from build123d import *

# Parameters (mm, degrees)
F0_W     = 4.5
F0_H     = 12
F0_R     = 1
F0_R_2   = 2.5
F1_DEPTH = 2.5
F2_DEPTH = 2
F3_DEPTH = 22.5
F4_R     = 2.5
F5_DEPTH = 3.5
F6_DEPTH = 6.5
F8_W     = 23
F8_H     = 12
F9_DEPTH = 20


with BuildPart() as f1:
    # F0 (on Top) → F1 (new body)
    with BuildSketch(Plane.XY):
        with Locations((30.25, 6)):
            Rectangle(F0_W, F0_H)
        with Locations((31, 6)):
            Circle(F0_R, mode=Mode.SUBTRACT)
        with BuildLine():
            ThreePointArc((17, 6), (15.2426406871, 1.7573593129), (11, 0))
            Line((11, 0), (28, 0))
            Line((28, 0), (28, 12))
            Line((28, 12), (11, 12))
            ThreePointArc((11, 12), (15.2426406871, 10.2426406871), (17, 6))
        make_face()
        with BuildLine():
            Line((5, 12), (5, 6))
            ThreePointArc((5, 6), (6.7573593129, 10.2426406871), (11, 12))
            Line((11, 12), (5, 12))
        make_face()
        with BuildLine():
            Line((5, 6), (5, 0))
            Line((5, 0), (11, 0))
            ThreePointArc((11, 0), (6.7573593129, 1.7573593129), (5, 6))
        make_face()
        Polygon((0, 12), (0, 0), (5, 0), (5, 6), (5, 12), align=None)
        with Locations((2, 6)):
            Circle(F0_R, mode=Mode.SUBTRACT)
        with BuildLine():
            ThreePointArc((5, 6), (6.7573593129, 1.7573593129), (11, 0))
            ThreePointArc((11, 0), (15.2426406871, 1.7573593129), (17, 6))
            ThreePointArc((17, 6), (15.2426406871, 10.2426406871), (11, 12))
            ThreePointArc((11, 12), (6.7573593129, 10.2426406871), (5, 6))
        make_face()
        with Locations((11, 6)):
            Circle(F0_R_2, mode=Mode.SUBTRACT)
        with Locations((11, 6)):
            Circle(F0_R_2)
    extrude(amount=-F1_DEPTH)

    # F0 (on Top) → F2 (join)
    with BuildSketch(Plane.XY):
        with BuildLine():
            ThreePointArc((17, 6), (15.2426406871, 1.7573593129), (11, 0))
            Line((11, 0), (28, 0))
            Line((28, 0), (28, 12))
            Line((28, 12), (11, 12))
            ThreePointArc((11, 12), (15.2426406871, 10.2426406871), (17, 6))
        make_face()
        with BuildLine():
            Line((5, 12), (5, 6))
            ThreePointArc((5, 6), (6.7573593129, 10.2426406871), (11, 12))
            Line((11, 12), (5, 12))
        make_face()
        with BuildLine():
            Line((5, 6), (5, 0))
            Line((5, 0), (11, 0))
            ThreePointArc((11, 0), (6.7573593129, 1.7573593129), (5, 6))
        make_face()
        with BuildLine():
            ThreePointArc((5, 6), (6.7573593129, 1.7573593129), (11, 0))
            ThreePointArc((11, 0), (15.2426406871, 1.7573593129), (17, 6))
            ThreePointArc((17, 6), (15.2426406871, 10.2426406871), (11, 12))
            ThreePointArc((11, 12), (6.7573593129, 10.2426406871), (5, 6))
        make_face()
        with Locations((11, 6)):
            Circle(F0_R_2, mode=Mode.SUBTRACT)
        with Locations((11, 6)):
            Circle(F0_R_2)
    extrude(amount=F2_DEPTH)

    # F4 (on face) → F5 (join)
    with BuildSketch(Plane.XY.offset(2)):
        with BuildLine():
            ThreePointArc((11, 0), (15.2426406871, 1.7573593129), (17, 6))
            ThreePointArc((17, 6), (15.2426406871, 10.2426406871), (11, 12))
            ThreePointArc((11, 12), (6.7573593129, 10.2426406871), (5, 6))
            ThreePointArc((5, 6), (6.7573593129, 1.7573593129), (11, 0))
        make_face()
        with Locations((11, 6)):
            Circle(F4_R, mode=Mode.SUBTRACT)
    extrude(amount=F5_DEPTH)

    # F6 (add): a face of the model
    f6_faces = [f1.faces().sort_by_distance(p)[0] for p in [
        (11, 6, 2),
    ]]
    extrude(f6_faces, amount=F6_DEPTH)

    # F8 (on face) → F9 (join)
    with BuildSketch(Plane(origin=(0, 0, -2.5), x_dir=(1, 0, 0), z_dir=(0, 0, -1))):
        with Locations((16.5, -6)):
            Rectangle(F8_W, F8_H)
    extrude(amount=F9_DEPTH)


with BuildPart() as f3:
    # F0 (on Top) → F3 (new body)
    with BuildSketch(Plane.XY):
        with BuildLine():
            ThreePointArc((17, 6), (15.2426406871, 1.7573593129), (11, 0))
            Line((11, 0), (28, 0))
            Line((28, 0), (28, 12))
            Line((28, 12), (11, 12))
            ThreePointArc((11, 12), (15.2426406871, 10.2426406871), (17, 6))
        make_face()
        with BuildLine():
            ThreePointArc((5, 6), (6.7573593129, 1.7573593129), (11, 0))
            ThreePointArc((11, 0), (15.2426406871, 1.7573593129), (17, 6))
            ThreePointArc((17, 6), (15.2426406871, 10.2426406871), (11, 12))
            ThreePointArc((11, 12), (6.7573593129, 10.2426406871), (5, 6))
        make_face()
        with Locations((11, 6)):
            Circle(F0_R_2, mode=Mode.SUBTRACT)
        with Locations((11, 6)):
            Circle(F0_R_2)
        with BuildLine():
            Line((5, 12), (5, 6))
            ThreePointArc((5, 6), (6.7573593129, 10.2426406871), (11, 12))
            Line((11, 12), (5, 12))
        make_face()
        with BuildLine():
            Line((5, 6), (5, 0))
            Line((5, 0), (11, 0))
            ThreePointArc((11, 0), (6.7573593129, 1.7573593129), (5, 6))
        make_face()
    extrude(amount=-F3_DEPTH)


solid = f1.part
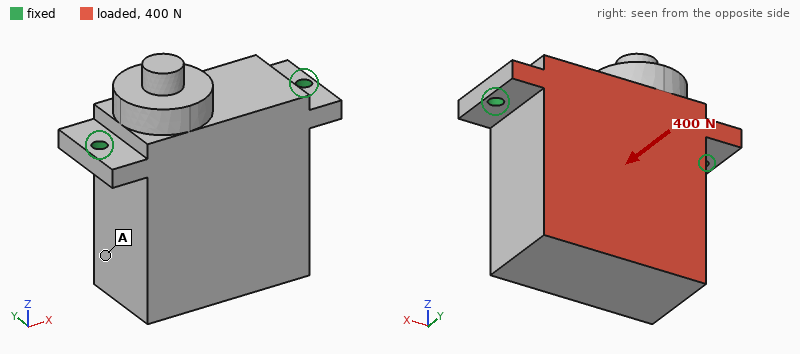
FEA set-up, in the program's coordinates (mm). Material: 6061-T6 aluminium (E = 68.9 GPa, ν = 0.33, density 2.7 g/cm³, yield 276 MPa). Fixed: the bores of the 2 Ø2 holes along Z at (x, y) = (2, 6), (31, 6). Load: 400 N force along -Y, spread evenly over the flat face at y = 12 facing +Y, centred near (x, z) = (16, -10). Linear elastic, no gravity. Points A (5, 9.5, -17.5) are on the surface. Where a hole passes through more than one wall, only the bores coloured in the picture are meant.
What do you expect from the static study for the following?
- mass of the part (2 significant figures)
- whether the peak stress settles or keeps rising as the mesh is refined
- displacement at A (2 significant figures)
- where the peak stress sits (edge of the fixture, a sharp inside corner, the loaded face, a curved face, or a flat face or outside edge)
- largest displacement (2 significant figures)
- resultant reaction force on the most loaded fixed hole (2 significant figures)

20 g
keeps rising
74 µm
edge of the fixture
98 µm
200 N
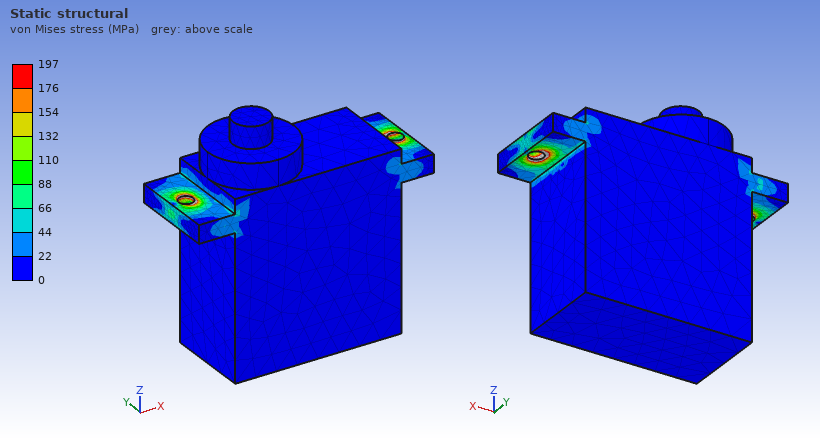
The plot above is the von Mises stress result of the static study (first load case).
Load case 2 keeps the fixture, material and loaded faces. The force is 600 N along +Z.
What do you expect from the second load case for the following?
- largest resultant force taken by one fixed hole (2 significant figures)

300 N
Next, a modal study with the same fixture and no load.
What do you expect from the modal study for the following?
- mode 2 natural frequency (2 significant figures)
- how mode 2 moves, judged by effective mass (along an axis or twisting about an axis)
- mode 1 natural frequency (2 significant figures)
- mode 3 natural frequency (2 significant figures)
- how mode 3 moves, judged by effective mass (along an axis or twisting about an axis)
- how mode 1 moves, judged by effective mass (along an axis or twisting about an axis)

12 kHz
along X
2700 Hz
13 kHz
along Z
along Y
